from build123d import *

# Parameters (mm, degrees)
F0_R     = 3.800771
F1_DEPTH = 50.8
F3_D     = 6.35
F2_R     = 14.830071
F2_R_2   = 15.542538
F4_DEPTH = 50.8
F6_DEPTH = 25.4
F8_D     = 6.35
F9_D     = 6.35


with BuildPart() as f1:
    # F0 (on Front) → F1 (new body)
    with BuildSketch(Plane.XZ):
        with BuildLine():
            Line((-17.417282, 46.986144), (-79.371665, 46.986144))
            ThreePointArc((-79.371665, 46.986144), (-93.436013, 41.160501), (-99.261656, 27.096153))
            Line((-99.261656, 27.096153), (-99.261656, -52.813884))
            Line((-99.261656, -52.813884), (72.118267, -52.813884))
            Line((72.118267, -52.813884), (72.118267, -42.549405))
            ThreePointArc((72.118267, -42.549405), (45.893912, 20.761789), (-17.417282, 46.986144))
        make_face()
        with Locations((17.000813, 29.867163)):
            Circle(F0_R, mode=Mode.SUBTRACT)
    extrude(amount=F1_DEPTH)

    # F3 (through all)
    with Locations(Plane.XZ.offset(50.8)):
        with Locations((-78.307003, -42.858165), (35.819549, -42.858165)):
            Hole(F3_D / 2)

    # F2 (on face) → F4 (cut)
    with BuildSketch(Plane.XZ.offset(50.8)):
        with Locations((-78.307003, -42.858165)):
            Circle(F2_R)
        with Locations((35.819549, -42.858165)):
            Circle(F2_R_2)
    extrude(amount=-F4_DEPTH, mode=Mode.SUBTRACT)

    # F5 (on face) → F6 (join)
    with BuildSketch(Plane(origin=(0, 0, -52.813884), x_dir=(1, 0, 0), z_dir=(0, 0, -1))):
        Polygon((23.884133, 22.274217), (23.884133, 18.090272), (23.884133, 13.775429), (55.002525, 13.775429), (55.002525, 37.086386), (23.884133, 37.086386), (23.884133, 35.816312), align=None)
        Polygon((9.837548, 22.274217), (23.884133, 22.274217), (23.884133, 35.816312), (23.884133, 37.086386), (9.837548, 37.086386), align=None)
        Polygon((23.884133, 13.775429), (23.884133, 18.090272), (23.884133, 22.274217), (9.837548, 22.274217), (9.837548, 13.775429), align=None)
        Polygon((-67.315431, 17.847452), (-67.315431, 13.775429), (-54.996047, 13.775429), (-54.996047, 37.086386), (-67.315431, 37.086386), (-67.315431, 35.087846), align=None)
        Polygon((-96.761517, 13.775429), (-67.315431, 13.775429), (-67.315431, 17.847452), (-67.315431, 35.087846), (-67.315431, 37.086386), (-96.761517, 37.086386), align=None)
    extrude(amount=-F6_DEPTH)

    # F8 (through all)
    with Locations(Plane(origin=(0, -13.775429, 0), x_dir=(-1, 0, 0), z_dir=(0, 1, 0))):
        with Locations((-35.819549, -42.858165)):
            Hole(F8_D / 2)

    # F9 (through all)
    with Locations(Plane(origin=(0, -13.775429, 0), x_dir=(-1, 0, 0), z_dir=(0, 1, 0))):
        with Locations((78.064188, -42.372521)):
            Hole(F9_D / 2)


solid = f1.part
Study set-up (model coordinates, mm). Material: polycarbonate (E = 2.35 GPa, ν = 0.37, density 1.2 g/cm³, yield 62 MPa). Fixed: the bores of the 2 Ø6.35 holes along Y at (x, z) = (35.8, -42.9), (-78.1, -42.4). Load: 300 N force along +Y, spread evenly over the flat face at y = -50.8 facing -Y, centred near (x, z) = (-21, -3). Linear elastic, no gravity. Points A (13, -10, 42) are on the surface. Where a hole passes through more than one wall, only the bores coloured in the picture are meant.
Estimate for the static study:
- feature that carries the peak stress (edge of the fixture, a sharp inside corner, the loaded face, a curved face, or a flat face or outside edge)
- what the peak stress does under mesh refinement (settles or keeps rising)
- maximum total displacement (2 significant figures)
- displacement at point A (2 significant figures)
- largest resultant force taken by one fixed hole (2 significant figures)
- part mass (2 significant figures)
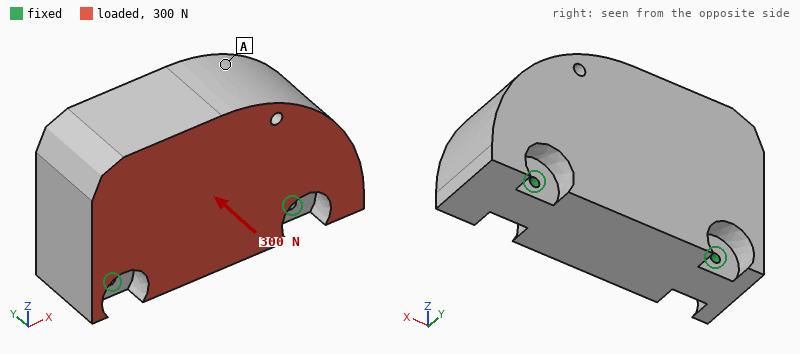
edge of the fixture
keeps rising
0.11 mm
0.097 mm
150 N
890 g
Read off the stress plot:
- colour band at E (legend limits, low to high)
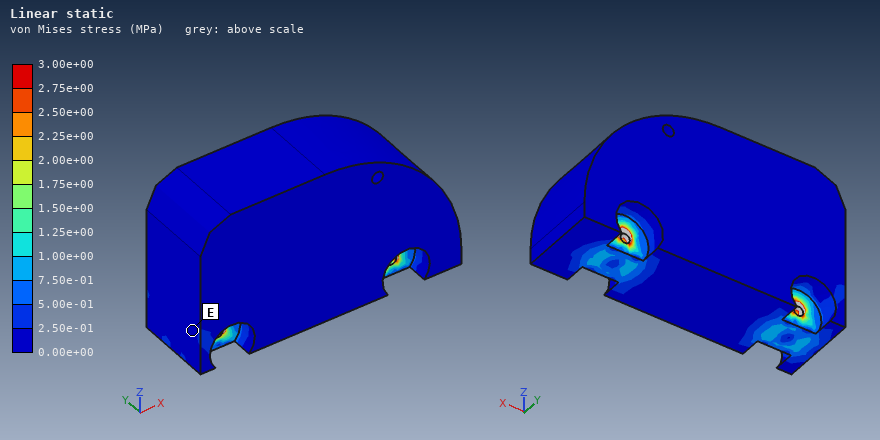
0.00e+00 to 2.50e-01 MPa
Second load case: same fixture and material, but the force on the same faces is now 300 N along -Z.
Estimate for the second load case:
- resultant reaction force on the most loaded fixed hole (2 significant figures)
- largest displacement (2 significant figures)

150 N
72 µm
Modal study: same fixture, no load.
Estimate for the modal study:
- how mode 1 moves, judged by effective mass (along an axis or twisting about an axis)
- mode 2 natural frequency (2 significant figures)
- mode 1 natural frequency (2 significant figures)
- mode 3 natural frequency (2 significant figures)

along Y
1300 Hz
350 Hz
1300 Hz
